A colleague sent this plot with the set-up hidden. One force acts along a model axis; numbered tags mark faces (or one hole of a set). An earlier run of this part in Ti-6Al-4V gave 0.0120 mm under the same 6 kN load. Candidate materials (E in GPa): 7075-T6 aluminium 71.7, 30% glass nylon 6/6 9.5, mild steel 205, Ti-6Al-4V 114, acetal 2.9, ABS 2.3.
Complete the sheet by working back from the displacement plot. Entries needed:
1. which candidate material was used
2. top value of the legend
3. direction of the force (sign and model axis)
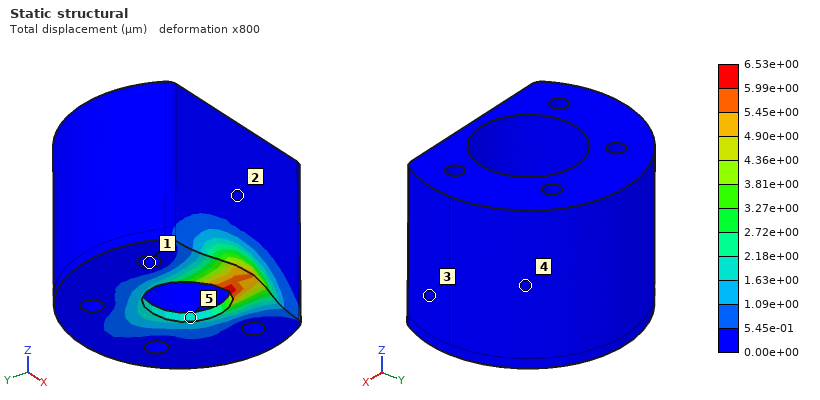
mild steel
6.53e+00 µm
-Y
